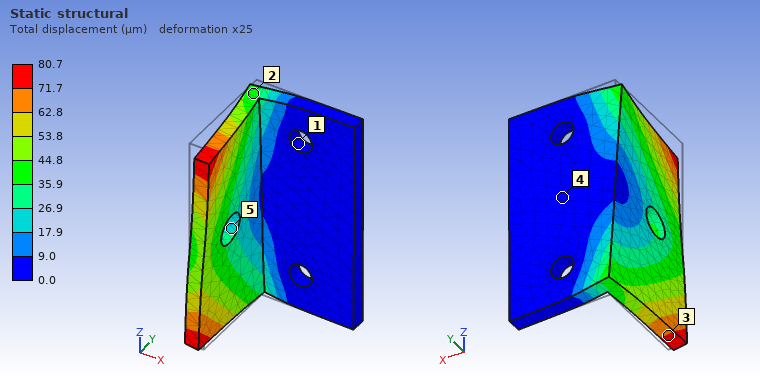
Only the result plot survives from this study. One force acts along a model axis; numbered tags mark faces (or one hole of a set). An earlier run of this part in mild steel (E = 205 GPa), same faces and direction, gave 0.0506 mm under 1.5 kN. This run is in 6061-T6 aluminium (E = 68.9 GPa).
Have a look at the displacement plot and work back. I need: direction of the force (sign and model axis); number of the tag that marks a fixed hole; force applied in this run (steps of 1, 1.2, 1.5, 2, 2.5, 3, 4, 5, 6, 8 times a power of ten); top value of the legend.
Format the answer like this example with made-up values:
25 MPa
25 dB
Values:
-Z
1
800 N
80.7 µm
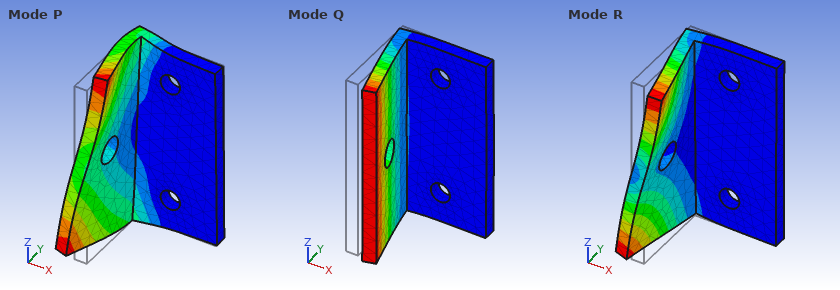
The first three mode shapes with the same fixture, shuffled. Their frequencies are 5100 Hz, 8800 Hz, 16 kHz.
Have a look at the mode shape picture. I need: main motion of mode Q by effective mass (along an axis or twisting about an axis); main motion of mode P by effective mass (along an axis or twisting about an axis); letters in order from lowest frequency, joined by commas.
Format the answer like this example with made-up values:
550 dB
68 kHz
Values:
along X
along Z
Q, R, P
